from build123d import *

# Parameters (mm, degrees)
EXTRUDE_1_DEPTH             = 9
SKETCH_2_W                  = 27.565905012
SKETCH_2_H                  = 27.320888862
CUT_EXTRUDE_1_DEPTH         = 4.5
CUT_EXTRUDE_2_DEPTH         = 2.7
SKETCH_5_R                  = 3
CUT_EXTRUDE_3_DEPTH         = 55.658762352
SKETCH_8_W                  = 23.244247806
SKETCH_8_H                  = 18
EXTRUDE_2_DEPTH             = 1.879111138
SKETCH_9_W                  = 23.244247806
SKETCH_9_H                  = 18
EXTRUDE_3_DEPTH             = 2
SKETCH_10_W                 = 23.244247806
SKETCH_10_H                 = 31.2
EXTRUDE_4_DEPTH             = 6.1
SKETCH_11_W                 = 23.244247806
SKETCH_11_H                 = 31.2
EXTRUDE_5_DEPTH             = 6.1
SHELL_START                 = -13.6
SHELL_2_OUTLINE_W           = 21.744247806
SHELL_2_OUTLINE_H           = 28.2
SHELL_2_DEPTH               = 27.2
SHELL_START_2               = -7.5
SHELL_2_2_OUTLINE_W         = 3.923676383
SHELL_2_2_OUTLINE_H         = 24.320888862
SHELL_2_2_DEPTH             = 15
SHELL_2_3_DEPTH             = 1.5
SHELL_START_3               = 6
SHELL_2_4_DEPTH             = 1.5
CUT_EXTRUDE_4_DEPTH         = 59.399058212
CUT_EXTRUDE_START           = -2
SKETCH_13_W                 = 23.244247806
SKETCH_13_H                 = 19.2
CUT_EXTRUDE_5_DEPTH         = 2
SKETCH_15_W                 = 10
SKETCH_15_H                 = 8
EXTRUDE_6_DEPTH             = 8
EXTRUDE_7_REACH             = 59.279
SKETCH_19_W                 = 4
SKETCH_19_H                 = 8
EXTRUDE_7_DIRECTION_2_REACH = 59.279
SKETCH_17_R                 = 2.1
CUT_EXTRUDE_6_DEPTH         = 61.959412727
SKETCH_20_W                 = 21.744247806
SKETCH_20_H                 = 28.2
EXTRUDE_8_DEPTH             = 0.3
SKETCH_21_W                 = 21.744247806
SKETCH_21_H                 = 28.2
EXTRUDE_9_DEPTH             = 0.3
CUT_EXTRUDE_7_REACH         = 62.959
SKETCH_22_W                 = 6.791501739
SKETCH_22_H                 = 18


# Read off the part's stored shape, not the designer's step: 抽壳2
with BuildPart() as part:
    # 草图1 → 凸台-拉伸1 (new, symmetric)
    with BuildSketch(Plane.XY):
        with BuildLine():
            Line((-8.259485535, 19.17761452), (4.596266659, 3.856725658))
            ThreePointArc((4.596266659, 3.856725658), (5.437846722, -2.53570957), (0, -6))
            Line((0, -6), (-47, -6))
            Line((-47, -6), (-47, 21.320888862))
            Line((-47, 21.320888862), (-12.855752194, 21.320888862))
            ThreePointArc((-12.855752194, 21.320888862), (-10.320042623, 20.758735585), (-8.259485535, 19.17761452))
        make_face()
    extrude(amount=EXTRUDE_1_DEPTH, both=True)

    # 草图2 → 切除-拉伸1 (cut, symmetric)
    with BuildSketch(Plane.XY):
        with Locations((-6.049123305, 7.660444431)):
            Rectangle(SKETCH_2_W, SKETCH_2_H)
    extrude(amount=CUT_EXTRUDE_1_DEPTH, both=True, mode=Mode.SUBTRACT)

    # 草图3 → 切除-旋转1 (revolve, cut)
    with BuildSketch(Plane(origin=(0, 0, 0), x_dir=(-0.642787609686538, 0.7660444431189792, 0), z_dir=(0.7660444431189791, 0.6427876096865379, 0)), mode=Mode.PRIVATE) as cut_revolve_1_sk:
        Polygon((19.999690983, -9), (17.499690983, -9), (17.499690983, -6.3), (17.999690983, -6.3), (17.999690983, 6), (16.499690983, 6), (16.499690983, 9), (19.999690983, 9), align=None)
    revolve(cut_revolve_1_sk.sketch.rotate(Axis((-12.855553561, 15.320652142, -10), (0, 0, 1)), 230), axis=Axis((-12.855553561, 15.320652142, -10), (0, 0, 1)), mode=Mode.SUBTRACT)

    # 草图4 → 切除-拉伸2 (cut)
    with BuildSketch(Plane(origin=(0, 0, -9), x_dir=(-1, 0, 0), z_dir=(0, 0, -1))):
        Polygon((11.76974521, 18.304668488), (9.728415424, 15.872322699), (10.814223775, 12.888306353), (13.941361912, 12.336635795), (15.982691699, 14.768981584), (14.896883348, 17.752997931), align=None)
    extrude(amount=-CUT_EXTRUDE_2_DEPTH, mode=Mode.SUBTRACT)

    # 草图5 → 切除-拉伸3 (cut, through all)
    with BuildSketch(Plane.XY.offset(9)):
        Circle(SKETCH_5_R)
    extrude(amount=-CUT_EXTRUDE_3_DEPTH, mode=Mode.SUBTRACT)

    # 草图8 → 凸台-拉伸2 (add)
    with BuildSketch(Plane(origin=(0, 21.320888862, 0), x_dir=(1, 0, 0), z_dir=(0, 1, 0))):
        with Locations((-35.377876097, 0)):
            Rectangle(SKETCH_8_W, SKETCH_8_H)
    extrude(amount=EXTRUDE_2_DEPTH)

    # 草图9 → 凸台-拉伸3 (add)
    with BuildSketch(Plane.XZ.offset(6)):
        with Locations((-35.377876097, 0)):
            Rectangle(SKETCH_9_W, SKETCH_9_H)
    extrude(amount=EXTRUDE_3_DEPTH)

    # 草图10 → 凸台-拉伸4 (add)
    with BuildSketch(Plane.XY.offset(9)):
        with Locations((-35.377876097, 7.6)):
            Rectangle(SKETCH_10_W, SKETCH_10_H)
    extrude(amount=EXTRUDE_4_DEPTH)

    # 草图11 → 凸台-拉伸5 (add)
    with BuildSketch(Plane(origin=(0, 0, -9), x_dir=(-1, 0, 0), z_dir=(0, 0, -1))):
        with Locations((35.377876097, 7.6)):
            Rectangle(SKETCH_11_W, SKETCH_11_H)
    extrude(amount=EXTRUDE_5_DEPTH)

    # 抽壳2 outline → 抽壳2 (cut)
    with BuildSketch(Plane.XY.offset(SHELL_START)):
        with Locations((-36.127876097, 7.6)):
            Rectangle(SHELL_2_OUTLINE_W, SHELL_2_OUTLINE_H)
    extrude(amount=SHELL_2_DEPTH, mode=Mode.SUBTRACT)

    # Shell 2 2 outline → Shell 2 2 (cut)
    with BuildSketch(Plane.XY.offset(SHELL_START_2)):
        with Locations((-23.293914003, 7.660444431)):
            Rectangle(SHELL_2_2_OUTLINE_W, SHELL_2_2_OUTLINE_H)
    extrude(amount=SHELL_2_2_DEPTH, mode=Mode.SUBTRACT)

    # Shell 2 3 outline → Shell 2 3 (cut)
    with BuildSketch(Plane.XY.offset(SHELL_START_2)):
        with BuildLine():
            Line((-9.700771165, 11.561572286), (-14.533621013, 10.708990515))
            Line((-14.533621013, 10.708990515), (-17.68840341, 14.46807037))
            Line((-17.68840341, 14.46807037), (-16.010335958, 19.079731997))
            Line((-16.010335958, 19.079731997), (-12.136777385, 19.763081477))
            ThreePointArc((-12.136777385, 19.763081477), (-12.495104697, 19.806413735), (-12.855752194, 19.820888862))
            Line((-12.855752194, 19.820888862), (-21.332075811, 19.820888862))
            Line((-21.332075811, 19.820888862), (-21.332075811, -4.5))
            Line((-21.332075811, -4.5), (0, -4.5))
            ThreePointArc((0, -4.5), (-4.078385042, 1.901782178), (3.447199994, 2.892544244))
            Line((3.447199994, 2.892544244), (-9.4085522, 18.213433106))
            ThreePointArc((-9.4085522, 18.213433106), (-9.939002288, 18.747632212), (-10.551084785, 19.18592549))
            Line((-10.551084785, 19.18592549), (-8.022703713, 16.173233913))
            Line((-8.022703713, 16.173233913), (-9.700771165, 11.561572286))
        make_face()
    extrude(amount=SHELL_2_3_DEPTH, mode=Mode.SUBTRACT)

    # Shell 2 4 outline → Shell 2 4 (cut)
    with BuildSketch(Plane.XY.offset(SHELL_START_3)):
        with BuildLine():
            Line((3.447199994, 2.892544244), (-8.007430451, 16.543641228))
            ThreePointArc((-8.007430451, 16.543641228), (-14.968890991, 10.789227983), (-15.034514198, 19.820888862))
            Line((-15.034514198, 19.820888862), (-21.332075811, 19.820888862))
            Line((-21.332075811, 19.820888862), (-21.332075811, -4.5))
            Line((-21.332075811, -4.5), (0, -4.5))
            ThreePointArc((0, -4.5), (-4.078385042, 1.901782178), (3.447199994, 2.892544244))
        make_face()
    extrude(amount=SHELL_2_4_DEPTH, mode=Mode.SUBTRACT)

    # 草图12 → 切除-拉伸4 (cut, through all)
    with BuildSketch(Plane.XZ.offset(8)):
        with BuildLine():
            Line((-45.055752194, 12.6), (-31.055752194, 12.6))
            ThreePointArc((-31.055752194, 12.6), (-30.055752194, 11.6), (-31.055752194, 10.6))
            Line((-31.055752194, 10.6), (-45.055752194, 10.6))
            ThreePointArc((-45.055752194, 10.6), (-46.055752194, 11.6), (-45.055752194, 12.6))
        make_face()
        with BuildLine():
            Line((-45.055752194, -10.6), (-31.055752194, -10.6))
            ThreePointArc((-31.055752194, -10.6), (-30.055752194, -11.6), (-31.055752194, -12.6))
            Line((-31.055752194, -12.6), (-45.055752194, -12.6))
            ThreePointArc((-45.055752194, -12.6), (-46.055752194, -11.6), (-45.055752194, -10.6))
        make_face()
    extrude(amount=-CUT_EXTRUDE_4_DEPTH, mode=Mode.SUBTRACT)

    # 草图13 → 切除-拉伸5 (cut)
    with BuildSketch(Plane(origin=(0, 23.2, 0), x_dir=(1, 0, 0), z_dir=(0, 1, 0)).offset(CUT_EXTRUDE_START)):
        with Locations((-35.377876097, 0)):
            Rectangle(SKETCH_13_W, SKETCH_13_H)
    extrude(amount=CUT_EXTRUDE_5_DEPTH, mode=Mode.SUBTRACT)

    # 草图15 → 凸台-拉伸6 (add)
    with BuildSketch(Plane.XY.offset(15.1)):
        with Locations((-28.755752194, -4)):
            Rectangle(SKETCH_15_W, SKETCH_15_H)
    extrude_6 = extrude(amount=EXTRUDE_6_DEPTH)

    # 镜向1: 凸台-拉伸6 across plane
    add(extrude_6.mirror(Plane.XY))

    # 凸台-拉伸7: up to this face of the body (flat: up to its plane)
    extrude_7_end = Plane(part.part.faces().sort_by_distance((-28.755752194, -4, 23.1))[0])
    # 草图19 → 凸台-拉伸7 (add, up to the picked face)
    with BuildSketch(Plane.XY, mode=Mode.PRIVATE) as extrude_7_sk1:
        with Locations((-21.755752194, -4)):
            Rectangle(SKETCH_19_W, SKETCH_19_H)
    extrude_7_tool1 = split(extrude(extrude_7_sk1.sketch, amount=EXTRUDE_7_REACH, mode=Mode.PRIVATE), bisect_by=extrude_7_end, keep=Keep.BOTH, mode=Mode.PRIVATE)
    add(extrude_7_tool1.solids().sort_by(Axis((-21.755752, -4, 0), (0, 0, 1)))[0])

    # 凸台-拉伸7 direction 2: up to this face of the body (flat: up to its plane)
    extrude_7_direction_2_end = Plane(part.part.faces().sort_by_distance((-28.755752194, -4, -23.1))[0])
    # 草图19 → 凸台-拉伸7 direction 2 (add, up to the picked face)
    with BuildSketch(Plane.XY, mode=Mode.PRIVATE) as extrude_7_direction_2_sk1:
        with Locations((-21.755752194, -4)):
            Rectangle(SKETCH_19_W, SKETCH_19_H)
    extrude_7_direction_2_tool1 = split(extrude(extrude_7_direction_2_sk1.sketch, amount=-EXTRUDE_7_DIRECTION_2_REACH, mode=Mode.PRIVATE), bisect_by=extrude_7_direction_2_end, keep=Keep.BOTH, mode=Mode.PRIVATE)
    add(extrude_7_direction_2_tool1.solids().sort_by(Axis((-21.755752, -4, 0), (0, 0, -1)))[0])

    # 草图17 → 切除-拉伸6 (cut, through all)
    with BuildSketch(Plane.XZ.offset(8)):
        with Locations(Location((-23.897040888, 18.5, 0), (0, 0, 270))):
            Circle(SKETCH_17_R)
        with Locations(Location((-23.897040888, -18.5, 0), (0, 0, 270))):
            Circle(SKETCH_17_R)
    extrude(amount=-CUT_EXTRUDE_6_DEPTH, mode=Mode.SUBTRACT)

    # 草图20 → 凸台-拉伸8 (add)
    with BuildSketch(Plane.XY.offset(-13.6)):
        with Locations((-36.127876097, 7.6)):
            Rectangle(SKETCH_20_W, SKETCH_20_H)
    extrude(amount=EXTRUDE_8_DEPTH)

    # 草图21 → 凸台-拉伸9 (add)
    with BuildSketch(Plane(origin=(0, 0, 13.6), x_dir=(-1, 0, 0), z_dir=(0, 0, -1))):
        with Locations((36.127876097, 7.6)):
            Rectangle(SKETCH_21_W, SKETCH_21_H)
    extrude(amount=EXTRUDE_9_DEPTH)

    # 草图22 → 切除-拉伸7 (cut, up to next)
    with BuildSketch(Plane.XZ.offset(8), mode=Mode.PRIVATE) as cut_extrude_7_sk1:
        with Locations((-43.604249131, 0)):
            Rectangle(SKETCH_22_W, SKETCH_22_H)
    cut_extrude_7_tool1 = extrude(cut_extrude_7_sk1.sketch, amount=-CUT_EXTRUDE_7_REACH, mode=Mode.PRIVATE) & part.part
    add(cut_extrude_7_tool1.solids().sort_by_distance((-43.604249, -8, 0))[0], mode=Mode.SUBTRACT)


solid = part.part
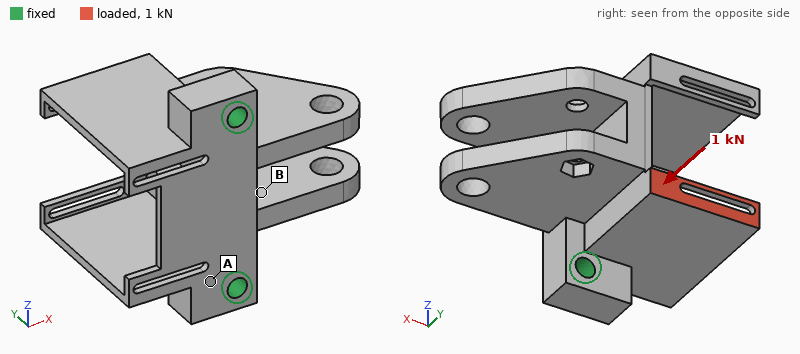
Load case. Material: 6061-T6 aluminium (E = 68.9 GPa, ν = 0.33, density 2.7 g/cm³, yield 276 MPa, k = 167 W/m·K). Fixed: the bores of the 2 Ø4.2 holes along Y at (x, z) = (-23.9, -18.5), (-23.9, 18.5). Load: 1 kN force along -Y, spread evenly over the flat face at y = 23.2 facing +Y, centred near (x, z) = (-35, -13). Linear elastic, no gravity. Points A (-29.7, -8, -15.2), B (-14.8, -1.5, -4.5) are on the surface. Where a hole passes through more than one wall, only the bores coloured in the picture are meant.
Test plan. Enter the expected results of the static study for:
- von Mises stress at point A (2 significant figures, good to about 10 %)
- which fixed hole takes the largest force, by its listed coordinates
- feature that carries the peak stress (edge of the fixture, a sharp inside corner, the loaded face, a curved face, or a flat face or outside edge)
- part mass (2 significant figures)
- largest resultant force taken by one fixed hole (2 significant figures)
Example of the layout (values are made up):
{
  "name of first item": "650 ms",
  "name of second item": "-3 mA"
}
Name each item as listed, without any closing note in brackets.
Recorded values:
{
  "von Mises stress at point A": "72 MPa",
  "which fixed hole takes the largest force, by its listed coordinates": "(-23.9, -18.5)",
  "feature that carries the peak stress": "a curved face",
  "part mass": "29 g",
  "largest resultant force taken by one fixed hole": "950 N"
}
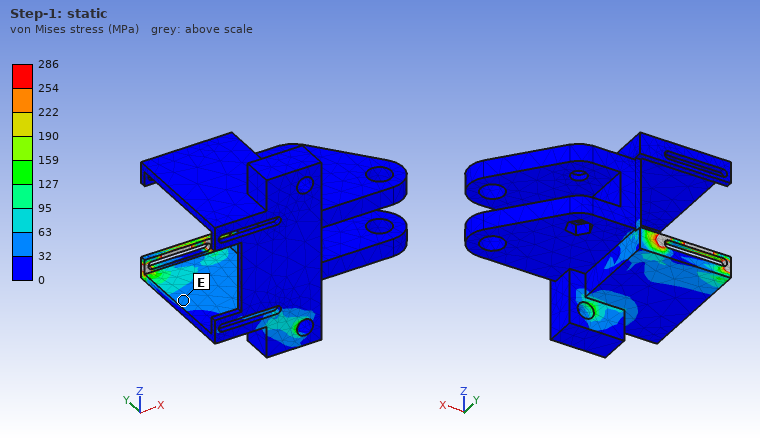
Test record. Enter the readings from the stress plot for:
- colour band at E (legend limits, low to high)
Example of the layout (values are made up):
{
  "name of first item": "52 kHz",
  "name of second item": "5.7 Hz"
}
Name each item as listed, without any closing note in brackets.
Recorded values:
{
  "colour band at E": "32 to 63 MPa"
}
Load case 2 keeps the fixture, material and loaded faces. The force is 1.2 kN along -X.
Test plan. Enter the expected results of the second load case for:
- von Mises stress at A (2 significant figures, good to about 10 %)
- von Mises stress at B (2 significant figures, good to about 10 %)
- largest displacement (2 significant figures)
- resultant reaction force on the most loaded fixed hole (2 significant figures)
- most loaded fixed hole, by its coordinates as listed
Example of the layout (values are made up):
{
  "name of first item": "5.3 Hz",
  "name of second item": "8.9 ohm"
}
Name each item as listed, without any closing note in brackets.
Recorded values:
{
  "von Mises stress at A": "190 MPa",
  "von Mises stress at B": "35 MPa",
  "largest displacement": "0.36 mm",
  "resultant reaction force on the most loaded fixed hole": "1.1 kN",
  "most loaded fixed hole, by its coordinates as listed": "(-23.9, -18.5)"
}
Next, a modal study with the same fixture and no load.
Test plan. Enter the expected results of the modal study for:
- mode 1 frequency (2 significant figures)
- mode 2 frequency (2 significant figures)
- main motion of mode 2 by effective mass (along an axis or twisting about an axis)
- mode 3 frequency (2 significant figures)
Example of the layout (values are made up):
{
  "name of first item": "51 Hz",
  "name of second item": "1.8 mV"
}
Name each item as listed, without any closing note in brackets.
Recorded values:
{
  "mode 1 frequency": "3300 Hz",
  "mode 2 frequency": "3700 Hz",
  "main motion of mode 2 by effective mass": "along Z",
  "mode 3 frequency": "4300 Hz"
}
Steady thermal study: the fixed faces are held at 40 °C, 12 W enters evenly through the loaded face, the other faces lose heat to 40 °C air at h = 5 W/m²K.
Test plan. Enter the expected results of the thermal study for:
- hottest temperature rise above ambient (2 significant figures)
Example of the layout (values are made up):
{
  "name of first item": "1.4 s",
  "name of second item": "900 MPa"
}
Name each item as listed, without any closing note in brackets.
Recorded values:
{
  "hottest temperature rise above ambient": "59 K"
}
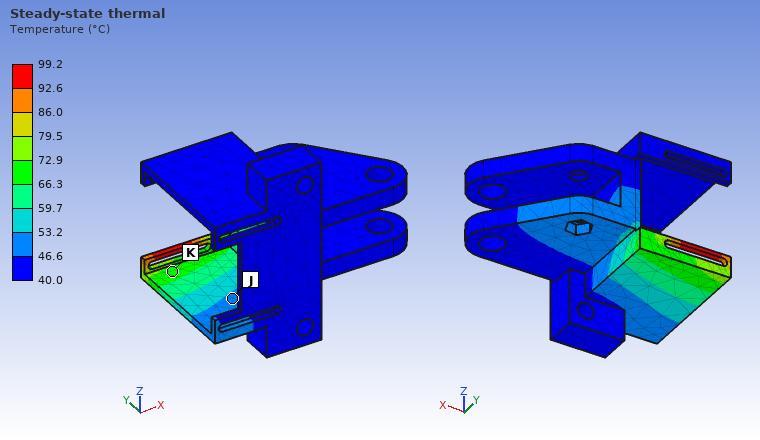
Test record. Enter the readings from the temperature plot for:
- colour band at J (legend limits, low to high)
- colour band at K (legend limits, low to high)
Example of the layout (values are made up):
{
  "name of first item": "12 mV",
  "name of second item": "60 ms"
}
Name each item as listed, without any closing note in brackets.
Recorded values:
{
  "colour band at J": "46.6 to 53.2 °C",
  "colour band at K": "66.3 to 72.9 °C"
}
